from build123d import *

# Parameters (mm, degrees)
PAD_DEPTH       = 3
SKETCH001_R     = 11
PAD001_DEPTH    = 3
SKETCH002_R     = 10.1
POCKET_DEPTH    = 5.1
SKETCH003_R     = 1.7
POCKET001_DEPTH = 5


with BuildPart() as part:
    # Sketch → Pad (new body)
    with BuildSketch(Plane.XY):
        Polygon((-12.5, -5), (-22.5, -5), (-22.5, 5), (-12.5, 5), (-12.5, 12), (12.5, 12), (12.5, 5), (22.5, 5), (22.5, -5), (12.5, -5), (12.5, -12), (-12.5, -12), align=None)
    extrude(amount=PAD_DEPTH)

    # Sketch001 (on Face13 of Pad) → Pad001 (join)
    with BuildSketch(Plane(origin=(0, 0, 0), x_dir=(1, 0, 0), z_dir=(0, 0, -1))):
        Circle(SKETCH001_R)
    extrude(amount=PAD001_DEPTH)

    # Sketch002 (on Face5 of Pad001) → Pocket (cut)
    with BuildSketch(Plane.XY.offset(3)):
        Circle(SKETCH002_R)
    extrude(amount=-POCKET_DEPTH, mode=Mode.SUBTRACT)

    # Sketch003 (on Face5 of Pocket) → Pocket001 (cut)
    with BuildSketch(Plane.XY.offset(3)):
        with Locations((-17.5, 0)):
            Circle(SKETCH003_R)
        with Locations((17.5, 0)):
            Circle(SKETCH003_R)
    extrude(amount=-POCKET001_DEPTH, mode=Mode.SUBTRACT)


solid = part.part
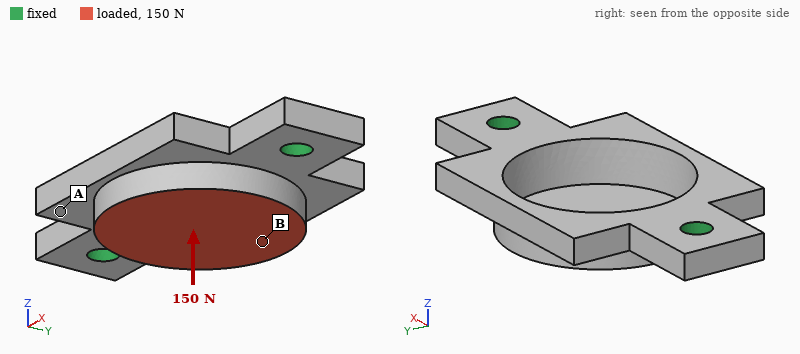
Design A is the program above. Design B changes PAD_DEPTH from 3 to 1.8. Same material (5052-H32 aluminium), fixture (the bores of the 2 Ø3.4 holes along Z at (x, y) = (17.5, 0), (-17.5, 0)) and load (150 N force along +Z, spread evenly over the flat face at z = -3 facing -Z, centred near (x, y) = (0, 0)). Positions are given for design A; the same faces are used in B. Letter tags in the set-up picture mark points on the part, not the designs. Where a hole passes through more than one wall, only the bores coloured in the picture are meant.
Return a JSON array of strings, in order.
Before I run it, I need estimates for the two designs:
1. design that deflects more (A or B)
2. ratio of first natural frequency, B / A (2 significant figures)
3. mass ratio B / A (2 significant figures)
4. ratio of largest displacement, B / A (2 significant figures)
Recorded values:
["B", "0.65", "0.70", "1.3"]
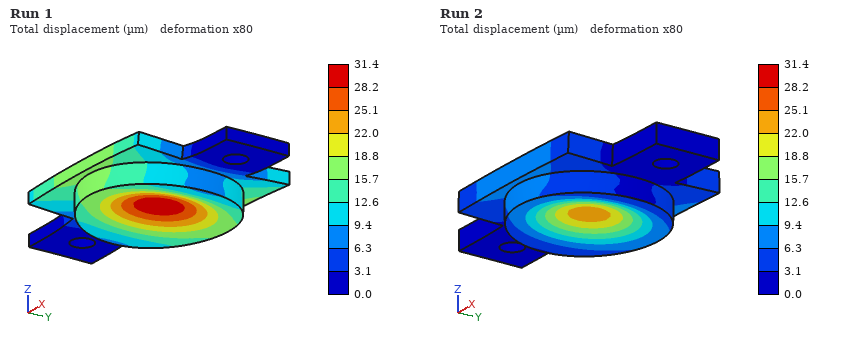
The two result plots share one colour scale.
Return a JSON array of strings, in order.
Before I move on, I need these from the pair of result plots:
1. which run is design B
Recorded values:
["Run 1"]
